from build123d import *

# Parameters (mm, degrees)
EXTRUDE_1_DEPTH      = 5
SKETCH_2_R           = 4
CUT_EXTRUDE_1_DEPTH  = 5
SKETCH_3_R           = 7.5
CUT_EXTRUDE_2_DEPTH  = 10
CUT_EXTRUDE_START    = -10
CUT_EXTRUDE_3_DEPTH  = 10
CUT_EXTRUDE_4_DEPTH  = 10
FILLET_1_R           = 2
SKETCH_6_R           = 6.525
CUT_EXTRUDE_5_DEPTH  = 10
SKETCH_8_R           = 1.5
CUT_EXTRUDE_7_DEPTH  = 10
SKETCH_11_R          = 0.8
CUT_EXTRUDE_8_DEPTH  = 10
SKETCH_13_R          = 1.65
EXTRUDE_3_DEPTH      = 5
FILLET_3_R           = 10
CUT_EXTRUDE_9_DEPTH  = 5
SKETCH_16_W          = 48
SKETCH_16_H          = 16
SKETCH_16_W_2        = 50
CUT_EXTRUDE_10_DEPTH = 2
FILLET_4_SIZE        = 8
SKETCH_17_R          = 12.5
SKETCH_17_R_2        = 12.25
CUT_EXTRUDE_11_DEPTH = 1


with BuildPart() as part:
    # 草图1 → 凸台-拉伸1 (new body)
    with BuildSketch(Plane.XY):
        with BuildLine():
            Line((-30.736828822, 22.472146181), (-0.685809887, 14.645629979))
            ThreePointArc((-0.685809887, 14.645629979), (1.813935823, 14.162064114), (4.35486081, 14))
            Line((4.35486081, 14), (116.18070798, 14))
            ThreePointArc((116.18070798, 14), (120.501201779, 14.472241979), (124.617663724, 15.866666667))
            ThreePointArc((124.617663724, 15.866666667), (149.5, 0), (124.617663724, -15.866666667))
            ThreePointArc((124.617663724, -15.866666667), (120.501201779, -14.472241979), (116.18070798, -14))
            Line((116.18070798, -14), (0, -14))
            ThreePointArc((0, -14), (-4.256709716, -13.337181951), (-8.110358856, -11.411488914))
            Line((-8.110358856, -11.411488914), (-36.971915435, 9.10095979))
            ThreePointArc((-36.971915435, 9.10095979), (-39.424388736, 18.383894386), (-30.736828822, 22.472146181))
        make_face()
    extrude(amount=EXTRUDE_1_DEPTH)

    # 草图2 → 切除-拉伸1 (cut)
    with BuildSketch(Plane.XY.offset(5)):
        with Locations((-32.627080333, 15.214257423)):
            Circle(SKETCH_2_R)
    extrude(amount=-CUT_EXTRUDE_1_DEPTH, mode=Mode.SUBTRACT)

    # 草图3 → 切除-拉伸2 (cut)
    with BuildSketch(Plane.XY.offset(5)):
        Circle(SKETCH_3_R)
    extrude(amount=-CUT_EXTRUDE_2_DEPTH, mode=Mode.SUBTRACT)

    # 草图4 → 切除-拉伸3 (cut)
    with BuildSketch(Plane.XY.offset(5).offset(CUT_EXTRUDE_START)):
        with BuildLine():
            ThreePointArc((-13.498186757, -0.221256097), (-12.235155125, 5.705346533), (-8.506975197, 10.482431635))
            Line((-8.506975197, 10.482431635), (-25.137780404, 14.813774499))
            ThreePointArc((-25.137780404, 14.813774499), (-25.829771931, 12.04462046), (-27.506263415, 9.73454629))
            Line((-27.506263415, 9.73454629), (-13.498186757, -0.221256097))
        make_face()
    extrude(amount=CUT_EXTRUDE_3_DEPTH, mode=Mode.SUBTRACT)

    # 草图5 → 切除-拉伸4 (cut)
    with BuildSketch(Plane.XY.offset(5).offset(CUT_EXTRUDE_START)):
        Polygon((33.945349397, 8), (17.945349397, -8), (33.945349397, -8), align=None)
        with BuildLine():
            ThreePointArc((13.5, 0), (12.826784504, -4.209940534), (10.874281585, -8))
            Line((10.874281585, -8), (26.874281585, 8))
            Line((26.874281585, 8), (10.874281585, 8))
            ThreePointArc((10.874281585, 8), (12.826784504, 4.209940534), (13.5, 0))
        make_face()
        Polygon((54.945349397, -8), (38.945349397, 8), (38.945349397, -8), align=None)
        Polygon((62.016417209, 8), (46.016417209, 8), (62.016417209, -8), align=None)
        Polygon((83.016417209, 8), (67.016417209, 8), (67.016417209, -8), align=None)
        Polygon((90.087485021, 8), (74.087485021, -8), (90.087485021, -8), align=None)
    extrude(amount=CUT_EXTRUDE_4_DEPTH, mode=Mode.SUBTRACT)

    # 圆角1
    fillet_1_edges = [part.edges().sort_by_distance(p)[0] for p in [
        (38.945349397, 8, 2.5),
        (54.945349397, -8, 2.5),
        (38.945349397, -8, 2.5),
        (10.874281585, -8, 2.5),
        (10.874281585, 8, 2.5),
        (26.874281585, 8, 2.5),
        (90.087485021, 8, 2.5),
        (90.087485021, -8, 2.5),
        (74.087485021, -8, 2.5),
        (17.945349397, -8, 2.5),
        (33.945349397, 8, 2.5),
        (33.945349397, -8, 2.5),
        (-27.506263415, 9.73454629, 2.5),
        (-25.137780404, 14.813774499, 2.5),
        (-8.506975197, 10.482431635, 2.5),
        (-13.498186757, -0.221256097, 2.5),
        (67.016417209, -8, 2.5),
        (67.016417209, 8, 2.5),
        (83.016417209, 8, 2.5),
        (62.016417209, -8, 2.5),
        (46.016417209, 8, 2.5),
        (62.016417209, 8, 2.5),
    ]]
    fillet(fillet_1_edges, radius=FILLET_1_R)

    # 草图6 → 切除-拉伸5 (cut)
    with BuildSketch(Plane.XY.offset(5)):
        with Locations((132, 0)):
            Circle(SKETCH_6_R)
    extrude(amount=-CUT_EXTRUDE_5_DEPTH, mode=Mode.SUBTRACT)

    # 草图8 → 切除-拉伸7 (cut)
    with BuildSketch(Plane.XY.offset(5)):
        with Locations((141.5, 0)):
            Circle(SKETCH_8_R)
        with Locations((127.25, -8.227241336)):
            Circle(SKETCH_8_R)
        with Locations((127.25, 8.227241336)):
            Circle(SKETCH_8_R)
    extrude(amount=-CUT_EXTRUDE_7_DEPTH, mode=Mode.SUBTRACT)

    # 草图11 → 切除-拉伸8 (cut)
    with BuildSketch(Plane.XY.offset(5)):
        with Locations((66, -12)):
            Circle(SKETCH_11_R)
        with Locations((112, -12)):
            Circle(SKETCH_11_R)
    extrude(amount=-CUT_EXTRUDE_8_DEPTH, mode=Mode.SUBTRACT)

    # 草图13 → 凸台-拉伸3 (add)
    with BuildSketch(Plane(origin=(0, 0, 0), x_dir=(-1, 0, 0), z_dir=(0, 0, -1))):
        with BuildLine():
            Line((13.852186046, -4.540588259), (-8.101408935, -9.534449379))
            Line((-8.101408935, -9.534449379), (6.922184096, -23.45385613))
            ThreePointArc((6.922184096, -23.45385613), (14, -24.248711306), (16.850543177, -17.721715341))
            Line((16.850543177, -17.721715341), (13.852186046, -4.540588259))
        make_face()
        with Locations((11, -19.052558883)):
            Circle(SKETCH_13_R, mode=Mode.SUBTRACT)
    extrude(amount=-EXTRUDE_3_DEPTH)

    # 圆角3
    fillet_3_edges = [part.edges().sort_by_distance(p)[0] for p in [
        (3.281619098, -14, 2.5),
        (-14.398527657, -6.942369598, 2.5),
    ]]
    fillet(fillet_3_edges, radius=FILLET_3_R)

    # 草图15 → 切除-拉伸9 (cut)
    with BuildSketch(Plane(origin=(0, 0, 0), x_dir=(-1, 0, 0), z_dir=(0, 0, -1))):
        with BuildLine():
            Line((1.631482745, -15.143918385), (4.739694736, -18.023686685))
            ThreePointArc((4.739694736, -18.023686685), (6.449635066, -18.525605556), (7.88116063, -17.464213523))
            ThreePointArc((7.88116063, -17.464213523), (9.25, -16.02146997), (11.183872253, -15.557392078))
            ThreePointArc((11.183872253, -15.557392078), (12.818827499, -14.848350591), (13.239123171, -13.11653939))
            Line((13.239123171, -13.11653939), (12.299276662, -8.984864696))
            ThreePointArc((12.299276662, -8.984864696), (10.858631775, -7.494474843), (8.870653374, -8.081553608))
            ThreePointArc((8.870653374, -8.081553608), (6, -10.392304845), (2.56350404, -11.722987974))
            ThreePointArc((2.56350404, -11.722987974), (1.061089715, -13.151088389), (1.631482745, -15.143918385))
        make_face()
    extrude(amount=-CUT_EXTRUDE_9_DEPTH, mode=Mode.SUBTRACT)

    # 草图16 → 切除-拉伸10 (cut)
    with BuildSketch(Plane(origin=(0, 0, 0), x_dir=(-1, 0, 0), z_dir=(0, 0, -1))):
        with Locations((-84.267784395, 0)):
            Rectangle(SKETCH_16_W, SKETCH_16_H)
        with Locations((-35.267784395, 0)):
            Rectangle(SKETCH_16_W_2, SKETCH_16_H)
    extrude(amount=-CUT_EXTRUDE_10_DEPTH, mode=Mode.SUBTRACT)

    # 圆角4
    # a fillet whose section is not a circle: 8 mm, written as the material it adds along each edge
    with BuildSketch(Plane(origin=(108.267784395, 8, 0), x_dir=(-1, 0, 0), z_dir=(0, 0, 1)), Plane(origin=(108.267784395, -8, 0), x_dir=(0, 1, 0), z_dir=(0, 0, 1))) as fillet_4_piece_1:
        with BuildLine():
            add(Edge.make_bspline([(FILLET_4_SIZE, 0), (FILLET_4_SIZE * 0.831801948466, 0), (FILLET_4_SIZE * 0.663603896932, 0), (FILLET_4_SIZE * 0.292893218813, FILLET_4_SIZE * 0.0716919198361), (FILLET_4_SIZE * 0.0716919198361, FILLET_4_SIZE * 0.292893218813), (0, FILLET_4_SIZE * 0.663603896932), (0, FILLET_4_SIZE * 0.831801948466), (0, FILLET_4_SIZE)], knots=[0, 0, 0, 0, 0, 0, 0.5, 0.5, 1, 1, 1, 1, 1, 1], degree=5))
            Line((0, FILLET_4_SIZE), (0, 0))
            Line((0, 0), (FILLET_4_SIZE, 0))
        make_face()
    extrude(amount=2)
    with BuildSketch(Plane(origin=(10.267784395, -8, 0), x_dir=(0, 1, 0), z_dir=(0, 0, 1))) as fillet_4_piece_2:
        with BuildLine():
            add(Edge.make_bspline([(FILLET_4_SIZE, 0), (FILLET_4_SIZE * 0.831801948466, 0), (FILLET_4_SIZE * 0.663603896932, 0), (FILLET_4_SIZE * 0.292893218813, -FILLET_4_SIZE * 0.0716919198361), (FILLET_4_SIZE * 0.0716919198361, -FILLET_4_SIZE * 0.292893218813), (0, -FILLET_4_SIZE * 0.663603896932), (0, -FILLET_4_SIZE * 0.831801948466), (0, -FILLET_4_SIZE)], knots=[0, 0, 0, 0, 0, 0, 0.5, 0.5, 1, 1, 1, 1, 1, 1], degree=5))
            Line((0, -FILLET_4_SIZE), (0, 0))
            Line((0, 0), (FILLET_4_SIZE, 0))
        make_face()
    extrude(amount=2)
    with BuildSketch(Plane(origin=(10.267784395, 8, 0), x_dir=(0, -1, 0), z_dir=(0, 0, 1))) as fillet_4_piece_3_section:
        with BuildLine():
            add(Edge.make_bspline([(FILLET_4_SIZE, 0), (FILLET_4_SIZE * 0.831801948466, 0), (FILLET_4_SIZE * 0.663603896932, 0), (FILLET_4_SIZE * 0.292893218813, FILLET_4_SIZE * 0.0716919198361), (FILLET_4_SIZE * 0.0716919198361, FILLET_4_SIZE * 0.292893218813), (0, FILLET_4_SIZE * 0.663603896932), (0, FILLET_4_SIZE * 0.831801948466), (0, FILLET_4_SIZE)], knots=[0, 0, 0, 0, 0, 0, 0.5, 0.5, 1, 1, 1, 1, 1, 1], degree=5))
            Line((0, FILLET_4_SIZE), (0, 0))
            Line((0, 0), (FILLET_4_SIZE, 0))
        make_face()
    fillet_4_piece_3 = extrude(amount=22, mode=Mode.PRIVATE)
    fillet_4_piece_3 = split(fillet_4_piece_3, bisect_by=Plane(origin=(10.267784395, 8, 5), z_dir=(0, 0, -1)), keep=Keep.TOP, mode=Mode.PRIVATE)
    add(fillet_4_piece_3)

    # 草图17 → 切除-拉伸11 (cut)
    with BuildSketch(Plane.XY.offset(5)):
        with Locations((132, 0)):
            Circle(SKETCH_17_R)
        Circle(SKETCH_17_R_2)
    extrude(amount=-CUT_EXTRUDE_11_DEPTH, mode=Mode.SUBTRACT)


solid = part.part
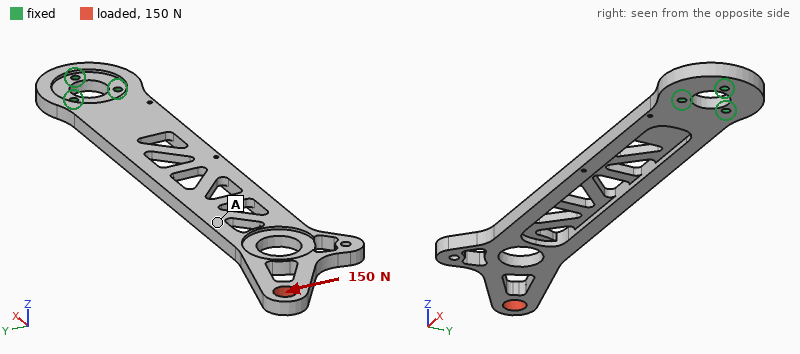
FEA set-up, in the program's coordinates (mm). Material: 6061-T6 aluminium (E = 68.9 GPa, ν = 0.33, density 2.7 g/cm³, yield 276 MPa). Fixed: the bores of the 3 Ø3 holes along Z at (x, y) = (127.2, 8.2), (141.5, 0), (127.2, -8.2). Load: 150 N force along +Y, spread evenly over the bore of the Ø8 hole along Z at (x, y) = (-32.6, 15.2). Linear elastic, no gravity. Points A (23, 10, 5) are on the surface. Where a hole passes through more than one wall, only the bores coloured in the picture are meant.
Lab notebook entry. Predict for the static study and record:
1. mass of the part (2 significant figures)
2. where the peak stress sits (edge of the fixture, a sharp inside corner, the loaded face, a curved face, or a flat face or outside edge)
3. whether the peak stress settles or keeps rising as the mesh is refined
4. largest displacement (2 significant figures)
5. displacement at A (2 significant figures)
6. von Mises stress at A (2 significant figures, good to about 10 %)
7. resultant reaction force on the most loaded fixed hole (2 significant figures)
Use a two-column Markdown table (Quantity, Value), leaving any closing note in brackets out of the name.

| Quantity | Value |
|---|---|
| mass of the part | 48 g |
| where the peak stress sits | edge of the fixture |
| whether the peak stress settles or keeps rising as the mesh is refined | keeps rising |
| largest displacement | 0.46 mm |
| displacement at A | 0.21 mm |
| von Mises stress at A | 7.0 MPa |
| resultant reaction force on the most loaded fixed hole | 1.2 kN |
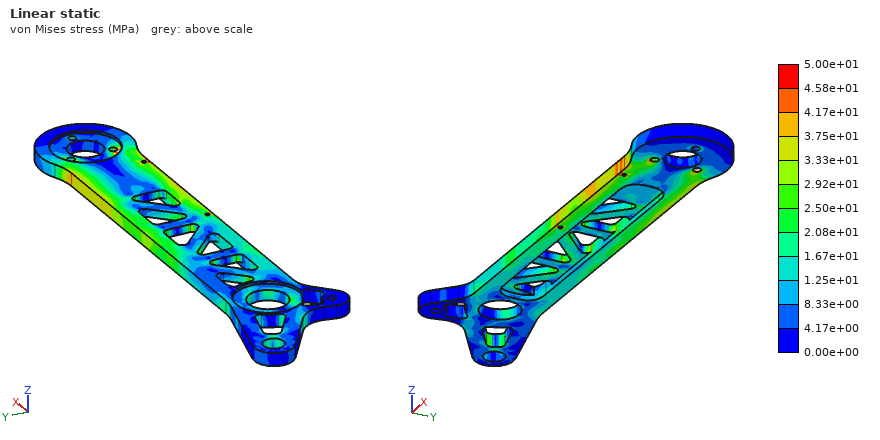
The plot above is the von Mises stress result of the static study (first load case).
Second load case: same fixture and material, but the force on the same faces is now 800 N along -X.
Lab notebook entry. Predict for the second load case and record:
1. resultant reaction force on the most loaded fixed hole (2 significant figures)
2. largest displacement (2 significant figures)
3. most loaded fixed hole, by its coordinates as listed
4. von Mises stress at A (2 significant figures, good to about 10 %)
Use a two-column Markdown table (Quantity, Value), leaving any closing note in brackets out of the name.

| Quantity | Value |
|---|---|
| resultant reaction force on the most loaded fixed hole | 980 N |
| largest displacement | 0.35 mm |
| most loaded fixed hole, by its coordinates as listed | (127.2, 8.2) |
| von Mises stress at A | 26 MPa |
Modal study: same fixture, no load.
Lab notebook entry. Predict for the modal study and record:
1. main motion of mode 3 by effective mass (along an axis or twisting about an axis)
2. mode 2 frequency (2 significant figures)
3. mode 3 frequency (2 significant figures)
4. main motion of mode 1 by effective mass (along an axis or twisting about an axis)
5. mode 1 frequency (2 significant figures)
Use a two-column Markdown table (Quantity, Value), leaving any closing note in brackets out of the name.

| Quantity | Value |
|---|---|
| main motion of mode 3 by effective mass | along Y |
| mode 2 frequency | 810 Hz |
| mode 3 frequency | 910 Hz |
| main motion of mode 1 by effective mass | along Z |
| mode 1 frequency | 150 Hz |
